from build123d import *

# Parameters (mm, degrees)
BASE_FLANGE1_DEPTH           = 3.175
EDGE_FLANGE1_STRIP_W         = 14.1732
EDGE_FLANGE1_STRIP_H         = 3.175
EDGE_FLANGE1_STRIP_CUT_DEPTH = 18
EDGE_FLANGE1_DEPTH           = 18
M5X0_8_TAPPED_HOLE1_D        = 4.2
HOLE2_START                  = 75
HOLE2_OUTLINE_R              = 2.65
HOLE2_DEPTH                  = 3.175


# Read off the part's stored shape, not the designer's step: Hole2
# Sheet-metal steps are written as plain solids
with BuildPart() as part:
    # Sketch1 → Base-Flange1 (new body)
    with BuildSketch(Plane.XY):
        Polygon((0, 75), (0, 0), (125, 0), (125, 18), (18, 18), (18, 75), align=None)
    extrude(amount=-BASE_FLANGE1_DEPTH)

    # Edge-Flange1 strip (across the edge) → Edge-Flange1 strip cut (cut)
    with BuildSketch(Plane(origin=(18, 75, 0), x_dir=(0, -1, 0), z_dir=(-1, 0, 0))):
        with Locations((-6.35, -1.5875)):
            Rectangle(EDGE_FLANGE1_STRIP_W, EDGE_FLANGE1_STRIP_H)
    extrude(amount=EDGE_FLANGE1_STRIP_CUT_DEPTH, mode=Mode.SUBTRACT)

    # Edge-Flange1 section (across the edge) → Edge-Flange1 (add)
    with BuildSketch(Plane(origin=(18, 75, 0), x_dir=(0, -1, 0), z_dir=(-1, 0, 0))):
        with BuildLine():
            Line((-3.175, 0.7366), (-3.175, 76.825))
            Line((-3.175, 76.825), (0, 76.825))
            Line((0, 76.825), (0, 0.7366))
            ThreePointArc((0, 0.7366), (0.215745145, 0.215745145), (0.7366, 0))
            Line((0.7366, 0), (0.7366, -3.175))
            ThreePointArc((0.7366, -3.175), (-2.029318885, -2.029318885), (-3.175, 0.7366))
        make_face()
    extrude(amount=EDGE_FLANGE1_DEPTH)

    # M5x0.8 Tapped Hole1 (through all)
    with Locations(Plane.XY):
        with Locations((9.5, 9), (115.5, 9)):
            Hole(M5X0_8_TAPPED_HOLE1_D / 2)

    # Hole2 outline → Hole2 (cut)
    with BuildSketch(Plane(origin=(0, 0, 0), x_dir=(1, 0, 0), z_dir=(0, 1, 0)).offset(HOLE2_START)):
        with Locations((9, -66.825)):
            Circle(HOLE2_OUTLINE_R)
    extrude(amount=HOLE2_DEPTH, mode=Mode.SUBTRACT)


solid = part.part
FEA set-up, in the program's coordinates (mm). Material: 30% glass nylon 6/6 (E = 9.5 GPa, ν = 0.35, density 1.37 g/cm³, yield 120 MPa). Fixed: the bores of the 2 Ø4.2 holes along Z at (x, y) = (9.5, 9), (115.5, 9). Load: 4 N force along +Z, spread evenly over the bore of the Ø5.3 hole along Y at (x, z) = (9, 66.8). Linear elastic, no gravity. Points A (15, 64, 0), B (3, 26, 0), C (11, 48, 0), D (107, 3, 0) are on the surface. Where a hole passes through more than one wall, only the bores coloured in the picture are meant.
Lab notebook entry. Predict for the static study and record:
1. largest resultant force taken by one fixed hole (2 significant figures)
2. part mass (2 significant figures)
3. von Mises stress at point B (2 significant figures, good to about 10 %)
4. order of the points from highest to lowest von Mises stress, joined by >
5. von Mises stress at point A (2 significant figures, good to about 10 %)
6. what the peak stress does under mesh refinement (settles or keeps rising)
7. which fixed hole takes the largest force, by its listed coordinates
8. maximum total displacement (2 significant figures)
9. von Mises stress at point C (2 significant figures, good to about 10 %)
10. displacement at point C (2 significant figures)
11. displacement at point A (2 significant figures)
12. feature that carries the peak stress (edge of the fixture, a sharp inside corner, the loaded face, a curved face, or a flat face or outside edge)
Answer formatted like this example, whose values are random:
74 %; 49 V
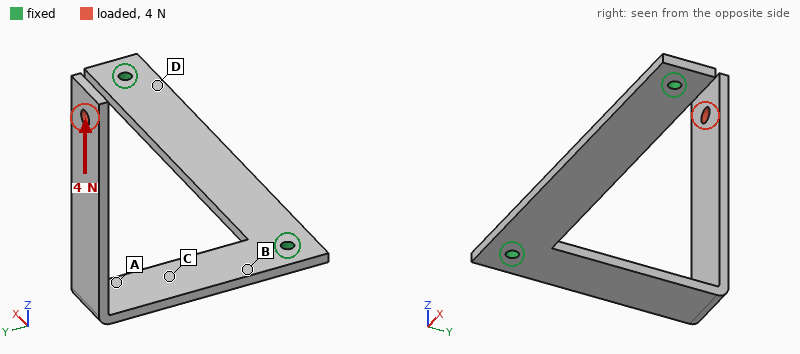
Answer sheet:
4.2 N; 20 g; 6.5 MPa; B > C > A > D; 1.7 MPa; keeps rising; (9.5, 9); 1.7 mm; 3.7 MPa; 0.34 mm; 0.60 mm; edge of the fixture
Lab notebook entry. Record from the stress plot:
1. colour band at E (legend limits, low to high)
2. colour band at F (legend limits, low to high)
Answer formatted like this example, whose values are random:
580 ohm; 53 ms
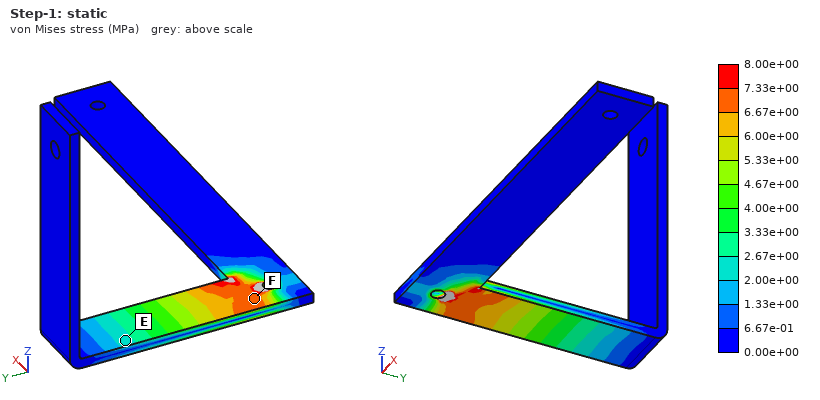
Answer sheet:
2.00e+00 to 2.67e+00 MPa; 6.67e+00 to 7.33e+00 MPa
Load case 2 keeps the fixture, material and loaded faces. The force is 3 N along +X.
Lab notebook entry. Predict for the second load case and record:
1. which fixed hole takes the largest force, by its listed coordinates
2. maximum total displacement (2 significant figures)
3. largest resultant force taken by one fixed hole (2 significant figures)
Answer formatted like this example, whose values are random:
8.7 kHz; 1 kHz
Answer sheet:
(9.5, 9); 1.7 mm; 2.4 N
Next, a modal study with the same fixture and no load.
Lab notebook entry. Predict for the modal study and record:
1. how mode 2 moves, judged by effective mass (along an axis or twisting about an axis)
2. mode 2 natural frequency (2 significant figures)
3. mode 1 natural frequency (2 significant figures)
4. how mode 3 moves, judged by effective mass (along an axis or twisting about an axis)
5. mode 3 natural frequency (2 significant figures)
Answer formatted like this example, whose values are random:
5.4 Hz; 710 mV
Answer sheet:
along X; 140 Hz; 88 Hz; along Z; 240 Hz
